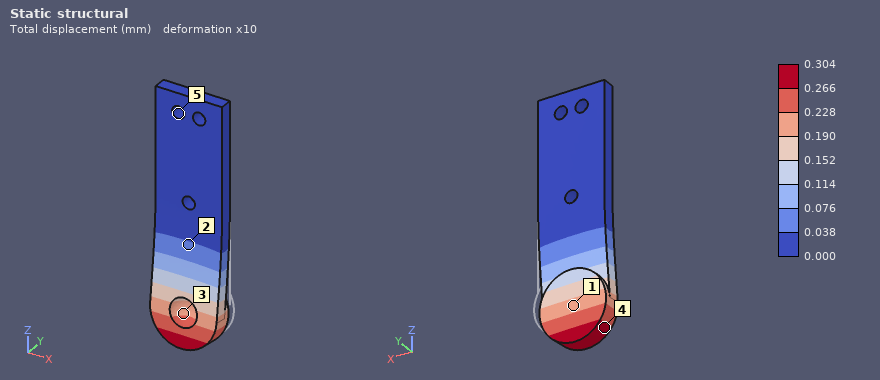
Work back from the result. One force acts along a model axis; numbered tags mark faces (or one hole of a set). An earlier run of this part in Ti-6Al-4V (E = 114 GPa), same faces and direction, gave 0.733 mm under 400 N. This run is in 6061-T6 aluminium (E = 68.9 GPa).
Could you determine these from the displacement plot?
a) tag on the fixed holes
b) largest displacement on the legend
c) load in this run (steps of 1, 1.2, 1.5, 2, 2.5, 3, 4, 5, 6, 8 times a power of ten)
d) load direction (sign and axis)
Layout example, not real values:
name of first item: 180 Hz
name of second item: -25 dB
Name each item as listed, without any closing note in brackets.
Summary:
tag on the fixed holes: 5
largest displacement on the legend: 0.304 mm
load in this run: 100 N
load direction: -Y
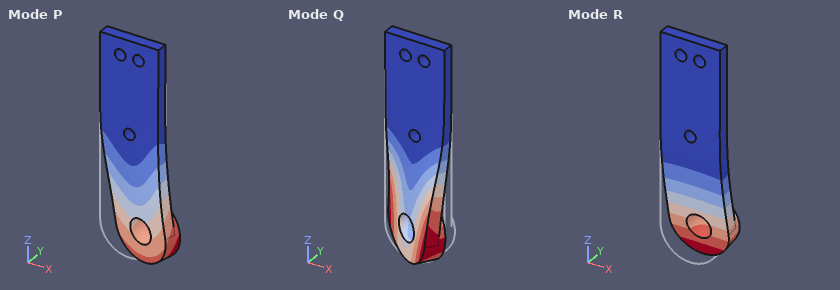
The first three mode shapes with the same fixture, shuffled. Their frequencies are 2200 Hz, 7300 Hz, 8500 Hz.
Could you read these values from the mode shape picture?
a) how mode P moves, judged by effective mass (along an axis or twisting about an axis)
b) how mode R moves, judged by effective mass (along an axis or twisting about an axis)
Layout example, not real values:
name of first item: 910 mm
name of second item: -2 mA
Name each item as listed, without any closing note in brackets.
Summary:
how mode P moves, judged by effective mass: along X
how mode R moves, judged by effective mass: along Y
